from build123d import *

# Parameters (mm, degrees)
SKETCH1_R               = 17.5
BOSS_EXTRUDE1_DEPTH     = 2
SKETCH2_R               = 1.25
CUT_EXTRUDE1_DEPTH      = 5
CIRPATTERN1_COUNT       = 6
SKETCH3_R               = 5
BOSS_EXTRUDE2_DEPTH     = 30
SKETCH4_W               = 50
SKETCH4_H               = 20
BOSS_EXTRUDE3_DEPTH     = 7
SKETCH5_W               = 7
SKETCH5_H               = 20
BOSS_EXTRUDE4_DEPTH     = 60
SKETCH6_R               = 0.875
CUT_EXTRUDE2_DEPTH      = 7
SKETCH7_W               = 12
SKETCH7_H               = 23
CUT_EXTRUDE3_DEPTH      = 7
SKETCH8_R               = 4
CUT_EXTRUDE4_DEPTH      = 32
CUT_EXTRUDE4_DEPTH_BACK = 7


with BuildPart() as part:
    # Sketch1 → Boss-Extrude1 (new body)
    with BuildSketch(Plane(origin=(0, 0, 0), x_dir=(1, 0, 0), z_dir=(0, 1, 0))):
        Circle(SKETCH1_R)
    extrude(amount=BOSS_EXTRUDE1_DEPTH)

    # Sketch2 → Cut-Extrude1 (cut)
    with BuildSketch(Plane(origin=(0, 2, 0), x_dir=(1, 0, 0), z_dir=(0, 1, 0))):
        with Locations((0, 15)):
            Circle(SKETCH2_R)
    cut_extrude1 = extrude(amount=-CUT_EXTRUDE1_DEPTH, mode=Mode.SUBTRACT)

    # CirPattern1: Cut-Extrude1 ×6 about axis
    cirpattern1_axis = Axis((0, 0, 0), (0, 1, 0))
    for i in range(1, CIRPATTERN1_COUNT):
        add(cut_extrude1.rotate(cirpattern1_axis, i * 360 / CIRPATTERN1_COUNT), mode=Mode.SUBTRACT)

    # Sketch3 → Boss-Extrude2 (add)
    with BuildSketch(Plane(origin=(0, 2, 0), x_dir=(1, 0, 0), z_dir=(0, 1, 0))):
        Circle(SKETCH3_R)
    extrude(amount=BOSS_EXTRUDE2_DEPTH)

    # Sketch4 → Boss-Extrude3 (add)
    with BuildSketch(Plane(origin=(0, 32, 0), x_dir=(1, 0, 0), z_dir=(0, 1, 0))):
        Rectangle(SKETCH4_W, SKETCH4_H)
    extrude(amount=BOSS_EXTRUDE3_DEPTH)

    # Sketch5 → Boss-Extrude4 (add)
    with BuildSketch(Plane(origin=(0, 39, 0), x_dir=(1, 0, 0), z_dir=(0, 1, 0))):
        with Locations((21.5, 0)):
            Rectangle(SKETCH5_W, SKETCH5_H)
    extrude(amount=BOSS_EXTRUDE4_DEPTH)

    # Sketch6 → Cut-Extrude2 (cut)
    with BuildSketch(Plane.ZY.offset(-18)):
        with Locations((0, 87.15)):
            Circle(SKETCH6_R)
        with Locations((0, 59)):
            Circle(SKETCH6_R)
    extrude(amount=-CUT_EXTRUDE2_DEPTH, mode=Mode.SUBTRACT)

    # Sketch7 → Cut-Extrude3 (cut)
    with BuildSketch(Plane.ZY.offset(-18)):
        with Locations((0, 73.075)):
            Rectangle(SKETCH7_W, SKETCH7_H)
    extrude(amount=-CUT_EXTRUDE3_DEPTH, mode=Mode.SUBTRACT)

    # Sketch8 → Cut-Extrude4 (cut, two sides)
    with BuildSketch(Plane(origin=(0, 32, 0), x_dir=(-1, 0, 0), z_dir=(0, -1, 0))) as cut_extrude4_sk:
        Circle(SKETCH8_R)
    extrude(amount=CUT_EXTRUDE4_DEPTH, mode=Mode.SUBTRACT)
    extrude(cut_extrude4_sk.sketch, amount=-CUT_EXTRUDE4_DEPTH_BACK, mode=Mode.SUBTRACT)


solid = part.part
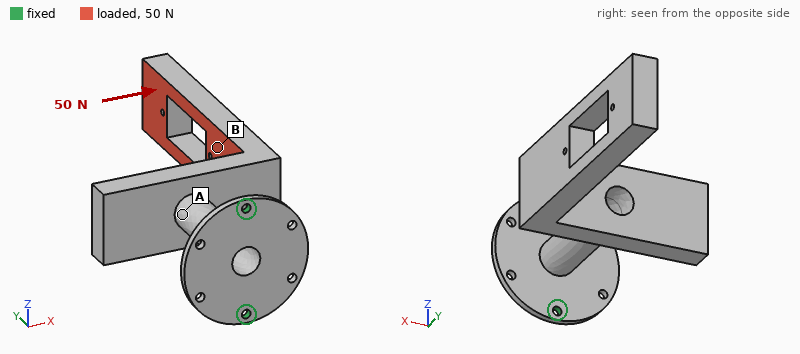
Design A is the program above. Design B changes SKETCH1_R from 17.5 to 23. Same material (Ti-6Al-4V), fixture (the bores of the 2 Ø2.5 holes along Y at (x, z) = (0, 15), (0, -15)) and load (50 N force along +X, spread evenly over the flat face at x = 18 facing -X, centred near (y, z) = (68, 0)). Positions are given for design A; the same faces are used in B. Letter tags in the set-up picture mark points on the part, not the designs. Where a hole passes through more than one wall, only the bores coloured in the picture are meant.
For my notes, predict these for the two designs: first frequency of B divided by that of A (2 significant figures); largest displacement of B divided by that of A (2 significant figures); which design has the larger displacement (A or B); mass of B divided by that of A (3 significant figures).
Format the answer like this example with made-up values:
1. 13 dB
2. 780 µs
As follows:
1. 1.1
2. 0.83
3. A
4. 1.09
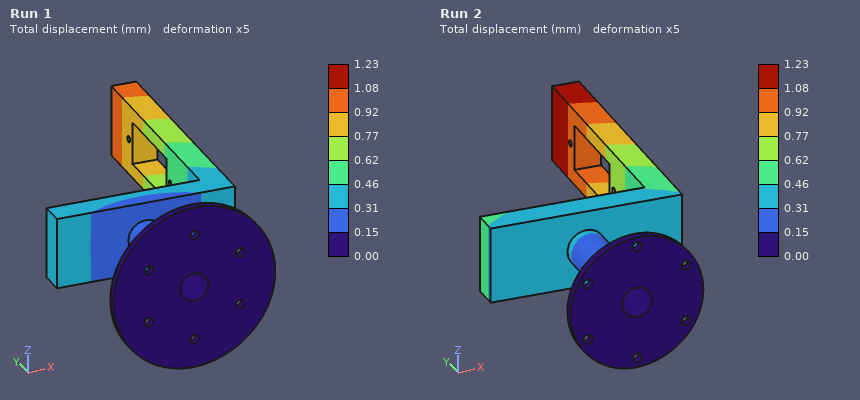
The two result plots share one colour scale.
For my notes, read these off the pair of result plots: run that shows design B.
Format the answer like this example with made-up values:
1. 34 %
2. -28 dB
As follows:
1. Run 1
